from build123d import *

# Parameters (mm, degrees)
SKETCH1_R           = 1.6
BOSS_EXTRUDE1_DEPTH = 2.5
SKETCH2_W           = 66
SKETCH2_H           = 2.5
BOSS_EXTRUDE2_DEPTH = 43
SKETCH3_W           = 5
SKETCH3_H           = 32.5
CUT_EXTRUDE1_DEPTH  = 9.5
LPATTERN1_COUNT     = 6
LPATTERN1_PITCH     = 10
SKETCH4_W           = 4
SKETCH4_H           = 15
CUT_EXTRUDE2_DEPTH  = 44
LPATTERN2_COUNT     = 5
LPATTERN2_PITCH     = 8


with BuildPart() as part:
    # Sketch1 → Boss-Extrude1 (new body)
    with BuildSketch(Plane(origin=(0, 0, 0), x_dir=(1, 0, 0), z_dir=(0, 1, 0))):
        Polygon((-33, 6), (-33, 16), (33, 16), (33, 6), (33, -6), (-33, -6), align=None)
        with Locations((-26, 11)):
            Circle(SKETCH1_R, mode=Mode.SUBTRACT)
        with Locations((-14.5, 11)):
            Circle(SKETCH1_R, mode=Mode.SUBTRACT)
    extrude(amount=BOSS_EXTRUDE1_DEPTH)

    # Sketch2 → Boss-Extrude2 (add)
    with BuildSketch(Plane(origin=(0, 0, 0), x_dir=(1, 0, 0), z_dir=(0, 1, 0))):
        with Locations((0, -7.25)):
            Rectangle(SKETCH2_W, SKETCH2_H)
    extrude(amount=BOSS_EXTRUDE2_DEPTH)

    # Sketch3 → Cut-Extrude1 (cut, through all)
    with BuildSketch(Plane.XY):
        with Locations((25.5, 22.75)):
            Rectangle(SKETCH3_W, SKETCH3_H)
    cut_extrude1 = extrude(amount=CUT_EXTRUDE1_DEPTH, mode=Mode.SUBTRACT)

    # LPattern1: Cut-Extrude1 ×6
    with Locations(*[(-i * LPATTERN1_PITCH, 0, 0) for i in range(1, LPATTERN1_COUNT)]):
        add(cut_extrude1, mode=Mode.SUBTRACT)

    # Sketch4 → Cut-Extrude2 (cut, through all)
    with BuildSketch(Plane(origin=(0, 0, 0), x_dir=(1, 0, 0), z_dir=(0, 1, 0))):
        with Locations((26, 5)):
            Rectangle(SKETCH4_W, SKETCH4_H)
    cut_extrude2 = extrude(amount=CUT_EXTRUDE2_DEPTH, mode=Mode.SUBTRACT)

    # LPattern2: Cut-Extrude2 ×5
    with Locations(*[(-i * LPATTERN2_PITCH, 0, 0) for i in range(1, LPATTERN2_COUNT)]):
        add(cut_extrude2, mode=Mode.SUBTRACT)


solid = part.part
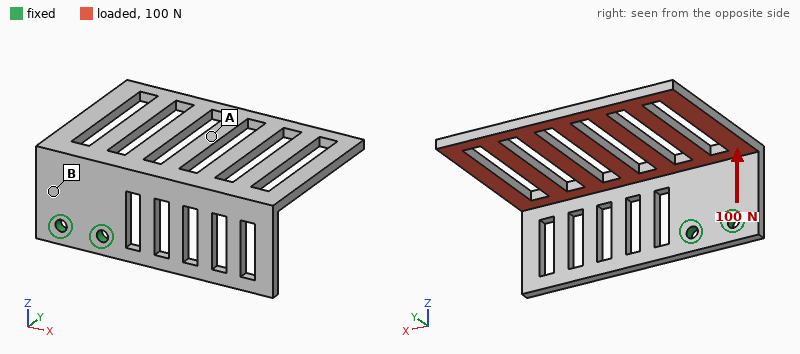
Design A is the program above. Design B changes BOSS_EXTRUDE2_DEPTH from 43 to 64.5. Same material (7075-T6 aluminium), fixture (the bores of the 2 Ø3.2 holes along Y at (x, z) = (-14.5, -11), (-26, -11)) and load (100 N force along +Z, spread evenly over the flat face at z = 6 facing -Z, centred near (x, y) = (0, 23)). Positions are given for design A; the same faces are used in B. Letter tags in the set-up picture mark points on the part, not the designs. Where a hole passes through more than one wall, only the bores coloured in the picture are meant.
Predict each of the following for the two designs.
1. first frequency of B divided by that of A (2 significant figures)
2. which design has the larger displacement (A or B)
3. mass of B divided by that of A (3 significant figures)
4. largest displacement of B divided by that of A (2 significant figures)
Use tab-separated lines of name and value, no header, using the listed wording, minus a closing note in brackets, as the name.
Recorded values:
first frequency of B divided by that of A	0.47
which design has the larger displacement	B
mass of B divided by that of A	1.47
largest displacement of B divided by that of A	2.7
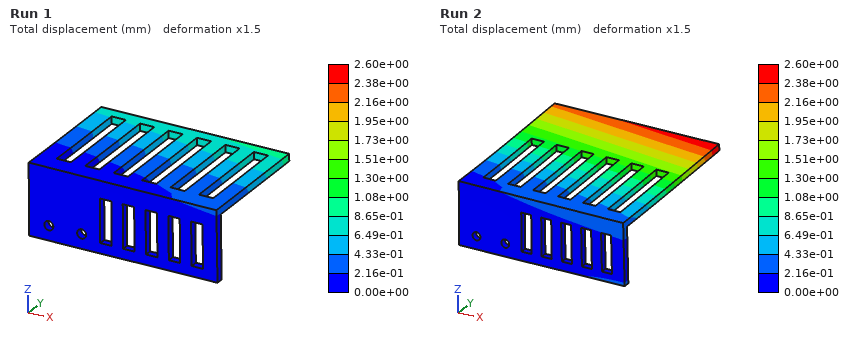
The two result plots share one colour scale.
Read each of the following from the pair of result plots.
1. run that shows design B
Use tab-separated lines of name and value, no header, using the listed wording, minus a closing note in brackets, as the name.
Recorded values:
run that shows design B	Run 2
